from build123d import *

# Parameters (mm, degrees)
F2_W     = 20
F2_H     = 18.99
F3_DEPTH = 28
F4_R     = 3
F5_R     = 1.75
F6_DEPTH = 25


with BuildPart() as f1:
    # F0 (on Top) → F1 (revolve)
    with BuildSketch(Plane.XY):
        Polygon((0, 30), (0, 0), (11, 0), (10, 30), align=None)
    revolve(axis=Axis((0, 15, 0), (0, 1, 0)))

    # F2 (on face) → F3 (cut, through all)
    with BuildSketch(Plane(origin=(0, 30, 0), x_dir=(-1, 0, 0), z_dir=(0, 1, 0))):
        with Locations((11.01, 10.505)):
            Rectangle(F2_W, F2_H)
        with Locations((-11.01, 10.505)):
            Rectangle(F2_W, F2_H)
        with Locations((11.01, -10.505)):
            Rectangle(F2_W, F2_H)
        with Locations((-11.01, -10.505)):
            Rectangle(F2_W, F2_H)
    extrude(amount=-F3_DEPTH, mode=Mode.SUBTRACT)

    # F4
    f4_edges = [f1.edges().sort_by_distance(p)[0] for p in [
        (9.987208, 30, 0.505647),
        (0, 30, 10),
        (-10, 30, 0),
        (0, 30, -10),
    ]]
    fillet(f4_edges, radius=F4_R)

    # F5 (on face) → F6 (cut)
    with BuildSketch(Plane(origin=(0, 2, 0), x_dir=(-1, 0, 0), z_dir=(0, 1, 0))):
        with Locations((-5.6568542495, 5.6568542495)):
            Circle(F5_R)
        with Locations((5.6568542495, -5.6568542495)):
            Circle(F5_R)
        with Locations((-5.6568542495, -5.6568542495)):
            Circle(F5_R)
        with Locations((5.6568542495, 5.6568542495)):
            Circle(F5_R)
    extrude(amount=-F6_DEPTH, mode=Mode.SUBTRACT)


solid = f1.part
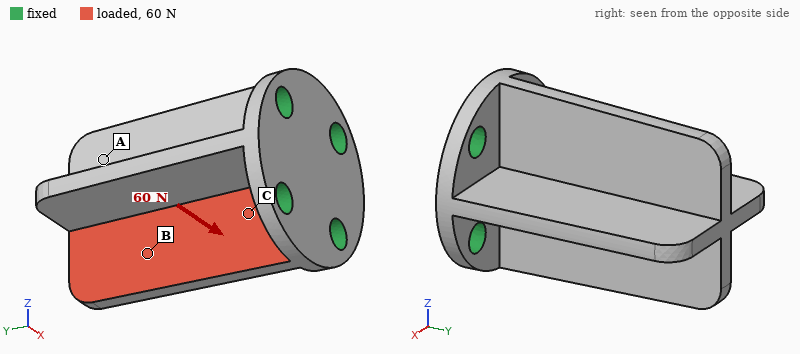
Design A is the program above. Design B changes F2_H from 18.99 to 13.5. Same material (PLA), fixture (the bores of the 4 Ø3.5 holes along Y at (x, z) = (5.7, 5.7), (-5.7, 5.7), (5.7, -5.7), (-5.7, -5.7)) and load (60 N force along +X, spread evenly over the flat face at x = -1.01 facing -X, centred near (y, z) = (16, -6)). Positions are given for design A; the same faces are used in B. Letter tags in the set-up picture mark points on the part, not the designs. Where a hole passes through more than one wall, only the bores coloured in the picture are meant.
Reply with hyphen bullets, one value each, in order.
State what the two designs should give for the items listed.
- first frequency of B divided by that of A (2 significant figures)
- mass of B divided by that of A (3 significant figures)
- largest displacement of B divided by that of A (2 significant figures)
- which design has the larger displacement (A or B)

- 1.1
- 1.96
- 0.20
- A
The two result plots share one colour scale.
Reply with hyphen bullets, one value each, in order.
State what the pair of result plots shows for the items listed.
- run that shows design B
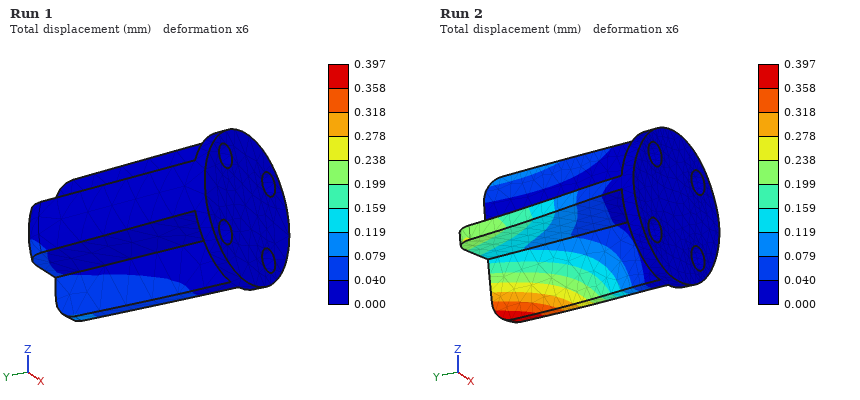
- Run 1
